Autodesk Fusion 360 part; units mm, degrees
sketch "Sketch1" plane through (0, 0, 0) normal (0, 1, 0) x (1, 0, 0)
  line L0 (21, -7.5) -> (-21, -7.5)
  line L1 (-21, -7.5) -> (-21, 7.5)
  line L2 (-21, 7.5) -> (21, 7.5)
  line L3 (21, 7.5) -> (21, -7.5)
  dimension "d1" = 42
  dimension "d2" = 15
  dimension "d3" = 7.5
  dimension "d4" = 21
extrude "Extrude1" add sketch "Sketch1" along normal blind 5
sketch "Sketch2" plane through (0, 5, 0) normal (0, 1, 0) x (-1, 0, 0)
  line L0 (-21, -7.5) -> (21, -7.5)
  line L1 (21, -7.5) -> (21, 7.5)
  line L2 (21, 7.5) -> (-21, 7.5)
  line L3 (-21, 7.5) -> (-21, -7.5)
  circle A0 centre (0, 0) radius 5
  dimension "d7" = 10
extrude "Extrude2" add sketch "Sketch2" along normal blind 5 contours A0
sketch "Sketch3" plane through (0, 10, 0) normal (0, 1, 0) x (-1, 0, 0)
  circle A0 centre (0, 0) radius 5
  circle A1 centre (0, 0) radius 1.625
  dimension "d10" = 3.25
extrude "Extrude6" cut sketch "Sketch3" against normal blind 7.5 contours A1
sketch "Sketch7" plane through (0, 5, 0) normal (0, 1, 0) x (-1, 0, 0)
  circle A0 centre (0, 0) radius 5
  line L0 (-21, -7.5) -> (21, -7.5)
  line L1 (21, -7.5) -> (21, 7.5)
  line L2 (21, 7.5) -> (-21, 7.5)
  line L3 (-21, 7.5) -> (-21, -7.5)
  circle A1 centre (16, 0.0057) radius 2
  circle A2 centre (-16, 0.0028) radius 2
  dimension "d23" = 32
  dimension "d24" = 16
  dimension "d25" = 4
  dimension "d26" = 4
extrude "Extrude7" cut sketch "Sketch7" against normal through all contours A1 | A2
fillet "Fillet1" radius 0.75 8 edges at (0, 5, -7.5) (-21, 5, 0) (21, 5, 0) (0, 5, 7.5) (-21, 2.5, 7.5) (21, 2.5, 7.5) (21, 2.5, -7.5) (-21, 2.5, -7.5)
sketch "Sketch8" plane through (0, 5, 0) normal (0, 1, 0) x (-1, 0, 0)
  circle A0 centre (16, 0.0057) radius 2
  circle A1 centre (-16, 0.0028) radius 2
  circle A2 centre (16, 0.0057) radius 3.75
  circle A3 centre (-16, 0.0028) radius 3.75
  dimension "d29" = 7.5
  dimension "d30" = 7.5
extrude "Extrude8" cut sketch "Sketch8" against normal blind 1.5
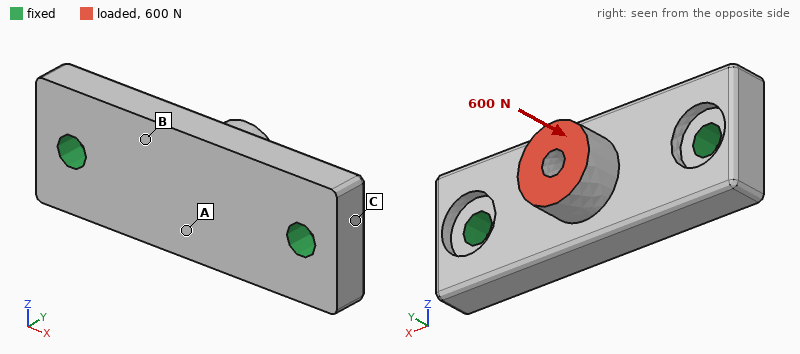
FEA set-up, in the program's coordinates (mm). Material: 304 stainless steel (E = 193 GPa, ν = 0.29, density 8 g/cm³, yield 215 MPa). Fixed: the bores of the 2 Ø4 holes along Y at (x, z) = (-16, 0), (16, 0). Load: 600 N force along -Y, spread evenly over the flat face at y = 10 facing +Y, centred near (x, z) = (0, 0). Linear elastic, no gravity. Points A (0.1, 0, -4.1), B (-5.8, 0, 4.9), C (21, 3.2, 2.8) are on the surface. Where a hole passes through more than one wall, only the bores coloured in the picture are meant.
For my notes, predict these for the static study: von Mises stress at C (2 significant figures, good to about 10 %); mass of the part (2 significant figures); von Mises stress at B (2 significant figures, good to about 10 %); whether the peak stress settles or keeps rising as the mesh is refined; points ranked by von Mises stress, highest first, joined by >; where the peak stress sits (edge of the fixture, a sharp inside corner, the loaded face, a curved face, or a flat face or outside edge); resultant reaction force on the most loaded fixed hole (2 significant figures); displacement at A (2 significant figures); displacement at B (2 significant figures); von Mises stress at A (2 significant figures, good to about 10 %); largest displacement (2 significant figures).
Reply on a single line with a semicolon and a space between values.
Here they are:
6.9 MPa; 26 g; 14 MPa; keeps rising; A > B > C; edge of the fixture; 350 N; 4.0 µm; 3.2 µm; 20 MPa; 4.1 µm
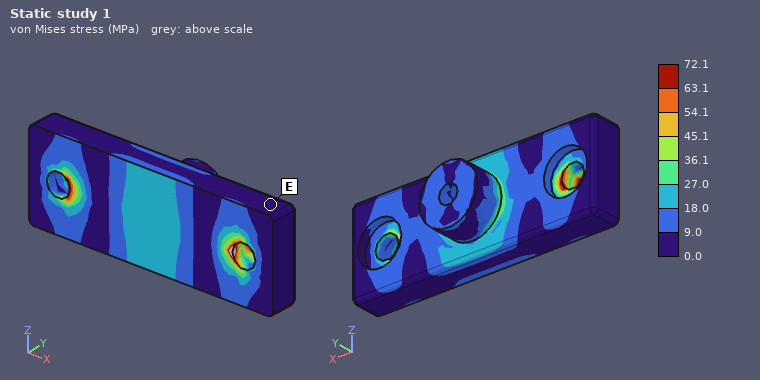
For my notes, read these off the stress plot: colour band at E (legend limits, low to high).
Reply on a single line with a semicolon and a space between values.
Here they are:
0.0 to 9.0 MPa
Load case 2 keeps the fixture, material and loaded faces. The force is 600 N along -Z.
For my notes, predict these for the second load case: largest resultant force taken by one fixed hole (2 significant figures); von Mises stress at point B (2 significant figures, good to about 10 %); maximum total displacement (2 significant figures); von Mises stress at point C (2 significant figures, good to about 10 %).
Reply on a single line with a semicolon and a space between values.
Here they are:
300 N; 23 MPa; 12 µm; 12 MPa
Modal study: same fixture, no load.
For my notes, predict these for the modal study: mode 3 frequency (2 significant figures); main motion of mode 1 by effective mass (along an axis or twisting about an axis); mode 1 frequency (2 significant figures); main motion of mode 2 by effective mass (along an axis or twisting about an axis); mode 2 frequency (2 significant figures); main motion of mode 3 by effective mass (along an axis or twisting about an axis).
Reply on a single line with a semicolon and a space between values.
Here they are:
29 kHz; along Y; 18 kHz; along Z; 19 kHz; along Z
